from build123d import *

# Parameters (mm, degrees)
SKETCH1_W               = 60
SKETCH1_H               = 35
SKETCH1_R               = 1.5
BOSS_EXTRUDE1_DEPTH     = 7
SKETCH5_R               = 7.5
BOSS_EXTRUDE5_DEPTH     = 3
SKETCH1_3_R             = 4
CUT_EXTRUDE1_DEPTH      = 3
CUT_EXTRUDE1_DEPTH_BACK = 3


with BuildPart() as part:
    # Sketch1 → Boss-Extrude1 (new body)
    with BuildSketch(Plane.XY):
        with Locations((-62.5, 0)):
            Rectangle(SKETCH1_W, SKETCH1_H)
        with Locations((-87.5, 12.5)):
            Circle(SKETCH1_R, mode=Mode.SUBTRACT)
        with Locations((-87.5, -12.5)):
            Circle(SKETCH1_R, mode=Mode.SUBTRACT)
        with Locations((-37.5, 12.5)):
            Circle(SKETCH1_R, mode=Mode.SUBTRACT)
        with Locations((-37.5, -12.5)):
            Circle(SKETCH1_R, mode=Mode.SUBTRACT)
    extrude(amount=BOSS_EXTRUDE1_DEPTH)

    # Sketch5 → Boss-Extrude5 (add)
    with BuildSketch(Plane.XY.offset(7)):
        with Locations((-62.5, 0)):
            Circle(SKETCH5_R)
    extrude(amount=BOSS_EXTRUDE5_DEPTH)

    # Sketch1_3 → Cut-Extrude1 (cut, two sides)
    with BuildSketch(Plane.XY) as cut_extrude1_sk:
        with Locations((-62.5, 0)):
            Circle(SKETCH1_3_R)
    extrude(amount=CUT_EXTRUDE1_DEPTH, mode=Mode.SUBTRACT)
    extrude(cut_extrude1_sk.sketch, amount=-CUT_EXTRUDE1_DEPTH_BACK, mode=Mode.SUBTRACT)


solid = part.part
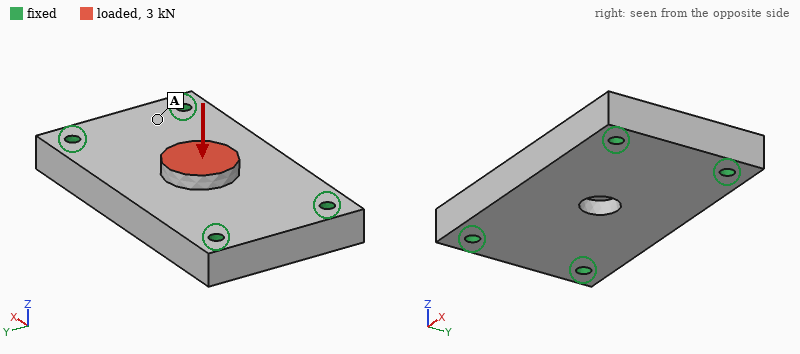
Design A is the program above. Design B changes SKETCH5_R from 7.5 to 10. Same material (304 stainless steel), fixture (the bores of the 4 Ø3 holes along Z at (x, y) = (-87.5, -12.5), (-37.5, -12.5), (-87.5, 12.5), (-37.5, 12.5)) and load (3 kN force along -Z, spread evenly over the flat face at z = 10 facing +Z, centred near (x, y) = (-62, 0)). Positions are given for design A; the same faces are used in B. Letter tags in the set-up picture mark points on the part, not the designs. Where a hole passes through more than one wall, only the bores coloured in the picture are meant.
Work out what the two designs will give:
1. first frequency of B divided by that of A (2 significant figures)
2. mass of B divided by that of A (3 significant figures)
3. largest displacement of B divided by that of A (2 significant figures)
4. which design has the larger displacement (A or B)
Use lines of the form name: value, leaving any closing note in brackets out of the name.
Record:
first frequency of B divided by that of A: 1.0
mass of B divided by that of A: 1.03
largest displacement of B divided by that of A: 0.85
which design has the larger displacement: A
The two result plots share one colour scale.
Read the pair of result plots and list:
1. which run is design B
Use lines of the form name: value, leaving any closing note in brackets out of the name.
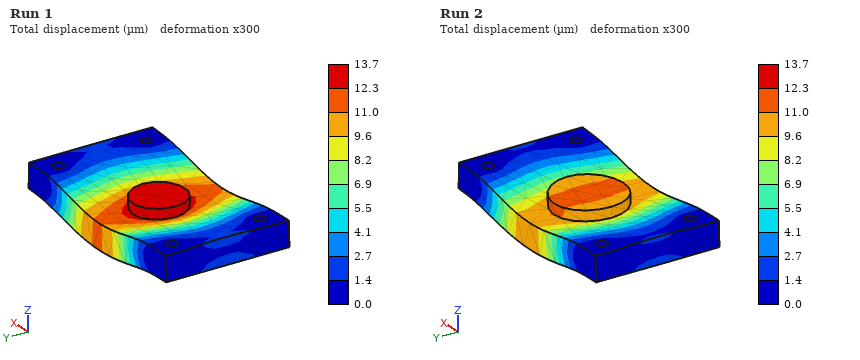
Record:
which run is design B: Run 2
